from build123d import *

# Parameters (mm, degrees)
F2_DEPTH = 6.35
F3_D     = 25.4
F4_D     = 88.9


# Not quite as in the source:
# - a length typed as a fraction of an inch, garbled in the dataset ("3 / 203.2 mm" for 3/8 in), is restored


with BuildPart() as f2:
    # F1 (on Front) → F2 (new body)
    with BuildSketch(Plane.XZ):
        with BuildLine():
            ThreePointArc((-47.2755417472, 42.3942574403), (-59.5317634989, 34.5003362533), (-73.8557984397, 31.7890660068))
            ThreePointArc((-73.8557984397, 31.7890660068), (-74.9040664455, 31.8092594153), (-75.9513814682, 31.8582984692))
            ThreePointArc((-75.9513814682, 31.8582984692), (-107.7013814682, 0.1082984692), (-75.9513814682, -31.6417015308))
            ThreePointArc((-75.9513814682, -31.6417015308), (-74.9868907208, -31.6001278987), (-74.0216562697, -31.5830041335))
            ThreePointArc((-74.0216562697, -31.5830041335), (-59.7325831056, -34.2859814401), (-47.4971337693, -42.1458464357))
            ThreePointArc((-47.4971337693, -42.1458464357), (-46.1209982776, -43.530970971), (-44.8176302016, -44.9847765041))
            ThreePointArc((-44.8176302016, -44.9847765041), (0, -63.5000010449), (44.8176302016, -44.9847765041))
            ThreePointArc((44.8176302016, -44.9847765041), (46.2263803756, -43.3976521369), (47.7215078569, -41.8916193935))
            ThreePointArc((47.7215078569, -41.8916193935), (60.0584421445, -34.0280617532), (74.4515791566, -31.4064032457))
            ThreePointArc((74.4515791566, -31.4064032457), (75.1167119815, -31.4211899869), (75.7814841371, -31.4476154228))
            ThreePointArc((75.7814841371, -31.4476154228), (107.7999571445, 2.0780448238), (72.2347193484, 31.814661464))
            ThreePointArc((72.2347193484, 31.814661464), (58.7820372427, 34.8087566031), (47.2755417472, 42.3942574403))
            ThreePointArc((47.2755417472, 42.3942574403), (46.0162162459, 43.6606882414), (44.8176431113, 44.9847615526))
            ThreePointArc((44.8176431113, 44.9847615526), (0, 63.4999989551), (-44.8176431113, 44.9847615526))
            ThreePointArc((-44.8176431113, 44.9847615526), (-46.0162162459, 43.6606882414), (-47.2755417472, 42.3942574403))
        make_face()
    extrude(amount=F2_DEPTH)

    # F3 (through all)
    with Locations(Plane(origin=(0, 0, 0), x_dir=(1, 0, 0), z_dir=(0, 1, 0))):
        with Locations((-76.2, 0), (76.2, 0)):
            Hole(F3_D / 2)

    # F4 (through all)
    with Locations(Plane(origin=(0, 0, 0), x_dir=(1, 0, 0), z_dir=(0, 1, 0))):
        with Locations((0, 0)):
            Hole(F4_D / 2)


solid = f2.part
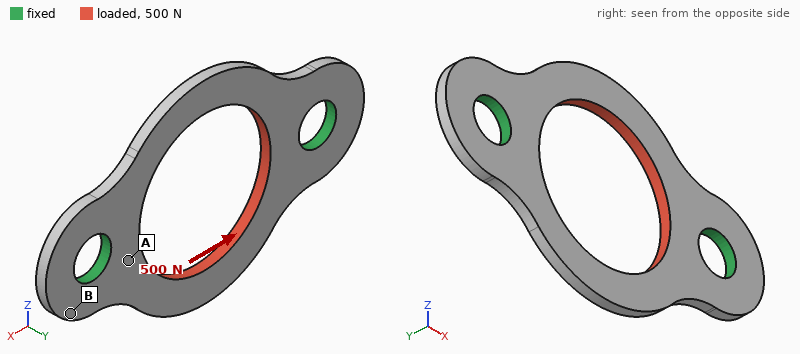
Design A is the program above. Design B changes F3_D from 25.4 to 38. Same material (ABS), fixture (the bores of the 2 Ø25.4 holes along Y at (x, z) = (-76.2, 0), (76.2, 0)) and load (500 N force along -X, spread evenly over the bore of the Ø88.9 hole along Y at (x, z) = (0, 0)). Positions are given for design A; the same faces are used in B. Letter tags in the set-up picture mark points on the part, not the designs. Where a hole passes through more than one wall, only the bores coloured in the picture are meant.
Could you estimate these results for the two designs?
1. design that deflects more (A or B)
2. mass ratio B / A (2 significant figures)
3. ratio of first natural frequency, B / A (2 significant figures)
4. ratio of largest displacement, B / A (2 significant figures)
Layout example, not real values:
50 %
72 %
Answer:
A
0.88
1.1
0.91
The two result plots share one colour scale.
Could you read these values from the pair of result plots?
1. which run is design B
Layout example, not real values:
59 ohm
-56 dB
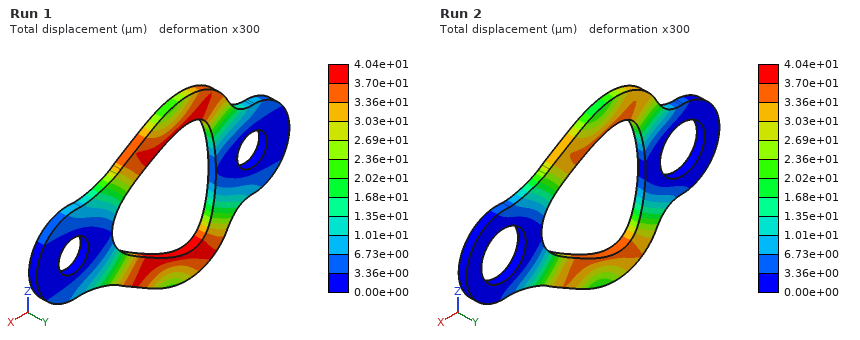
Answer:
Run 2
